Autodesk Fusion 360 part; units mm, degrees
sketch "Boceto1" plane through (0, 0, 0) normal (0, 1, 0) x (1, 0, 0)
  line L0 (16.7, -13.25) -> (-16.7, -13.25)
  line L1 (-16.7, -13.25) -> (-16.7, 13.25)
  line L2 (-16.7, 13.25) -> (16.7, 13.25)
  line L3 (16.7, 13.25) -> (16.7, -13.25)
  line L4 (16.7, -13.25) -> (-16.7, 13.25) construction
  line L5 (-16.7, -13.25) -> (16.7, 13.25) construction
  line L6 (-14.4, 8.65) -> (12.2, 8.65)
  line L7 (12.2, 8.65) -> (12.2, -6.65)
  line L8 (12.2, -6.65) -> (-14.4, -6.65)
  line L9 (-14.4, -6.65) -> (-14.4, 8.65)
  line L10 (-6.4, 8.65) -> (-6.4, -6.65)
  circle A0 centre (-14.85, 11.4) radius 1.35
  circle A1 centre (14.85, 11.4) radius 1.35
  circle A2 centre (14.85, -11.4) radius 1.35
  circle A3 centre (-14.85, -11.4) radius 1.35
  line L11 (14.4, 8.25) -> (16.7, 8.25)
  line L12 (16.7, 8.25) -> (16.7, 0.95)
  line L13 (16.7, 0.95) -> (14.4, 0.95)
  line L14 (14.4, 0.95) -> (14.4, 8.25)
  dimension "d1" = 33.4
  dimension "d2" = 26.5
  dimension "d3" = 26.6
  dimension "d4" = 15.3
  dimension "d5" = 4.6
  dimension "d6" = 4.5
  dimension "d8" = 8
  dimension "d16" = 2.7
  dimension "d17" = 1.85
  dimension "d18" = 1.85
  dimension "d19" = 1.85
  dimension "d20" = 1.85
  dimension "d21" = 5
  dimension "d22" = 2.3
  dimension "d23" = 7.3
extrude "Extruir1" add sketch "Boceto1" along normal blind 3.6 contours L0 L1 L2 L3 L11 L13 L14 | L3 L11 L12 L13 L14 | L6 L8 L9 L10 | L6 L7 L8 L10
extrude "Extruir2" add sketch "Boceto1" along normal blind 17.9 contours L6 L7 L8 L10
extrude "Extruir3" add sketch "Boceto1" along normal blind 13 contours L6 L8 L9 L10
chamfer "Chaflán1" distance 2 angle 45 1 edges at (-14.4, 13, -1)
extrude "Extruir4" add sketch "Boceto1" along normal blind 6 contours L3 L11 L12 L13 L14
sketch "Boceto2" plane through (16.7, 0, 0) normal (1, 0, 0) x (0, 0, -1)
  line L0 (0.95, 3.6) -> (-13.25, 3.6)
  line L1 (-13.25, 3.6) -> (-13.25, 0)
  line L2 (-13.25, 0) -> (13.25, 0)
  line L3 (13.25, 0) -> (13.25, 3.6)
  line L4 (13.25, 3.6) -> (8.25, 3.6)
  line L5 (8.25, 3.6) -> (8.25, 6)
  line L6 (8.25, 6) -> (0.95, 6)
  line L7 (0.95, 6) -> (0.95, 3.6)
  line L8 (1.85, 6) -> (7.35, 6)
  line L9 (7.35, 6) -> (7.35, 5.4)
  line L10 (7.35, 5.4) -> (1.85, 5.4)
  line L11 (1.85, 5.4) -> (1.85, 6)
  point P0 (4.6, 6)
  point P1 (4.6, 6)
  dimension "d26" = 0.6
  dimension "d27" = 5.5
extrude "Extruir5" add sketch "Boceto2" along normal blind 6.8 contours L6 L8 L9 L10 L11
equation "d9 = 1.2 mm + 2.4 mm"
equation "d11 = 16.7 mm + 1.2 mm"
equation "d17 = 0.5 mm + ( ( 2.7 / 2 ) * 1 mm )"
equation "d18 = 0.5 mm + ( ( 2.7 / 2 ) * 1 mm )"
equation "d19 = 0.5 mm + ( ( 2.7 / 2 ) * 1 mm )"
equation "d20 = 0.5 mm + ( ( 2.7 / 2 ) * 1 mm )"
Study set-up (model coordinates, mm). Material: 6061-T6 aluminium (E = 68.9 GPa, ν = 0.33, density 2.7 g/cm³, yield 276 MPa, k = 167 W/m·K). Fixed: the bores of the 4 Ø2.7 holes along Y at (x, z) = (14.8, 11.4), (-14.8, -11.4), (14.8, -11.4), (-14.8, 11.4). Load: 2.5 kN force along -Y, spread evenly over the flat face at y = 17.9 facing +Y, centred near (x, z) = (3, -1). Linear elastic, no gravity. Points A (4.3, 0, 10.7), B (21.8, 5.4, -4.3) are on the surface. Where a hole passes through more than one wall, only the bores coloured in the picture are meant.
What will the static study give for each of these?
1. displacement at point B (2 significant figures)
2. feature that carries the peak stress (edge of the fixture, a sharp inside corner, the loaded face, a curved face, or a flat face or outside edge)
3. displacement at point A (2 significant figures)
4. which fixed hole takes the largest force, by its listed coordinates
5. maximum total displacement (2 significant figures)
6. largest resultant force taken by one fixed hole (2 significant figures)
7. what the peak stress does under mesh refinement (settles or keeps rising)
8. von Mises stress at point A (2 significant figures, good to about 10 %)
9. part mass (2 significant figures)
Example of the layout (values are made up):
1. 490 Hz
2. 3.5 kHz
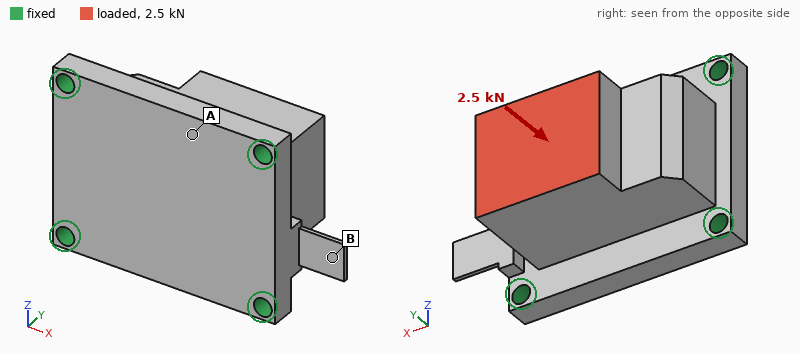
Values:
1. 6.6 µm
2. edge of the fixture
3. 14 µm
4. (14.8, -11.4)
5. 22 µm
6. 900 N
7. keeps rising
8. 31 MPa
9. 23 g
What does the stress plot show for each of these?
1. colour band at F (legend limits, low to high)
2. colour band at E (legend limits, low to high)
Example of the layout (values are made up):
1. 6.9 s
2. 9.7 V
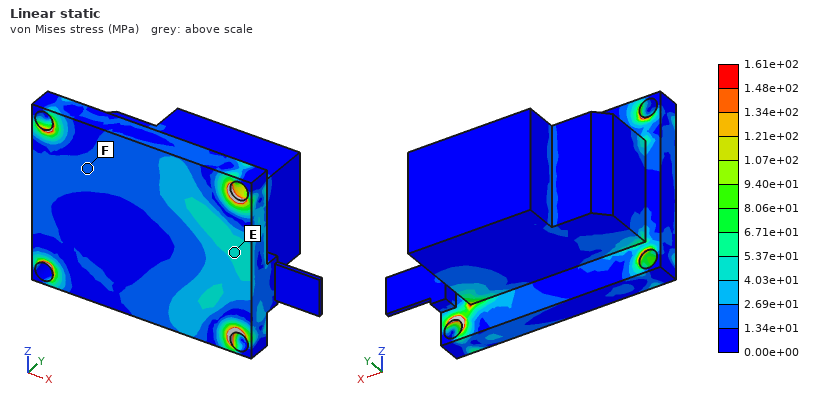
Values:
1. 1.34e+01 to 2.69e+01 MPa
2. 4.03e+01 to 5.37e+01 MPa
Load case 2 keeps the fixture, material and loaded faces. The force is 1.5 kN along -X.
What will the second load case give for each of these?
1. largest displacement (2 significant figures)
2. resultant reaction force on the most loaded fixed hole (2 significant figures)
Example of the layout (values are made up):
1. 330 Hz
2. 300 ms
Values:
1. 20 µm
2. 760 N
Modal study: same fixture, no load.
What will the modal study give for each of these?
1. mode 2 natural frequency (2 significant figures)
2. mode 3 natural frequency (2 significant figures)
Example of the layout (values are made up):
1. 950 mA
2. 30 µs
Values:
1. 14 kHz
2. 16 kHz
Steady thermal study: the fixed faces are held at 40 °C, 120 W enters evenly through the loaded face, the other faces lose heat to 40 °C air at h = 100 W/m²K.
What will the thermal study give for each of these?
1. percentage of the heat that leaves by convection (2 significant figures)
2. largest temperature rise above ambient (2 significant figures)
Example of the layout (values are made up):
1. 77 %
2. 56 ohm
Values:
1. 8.8 %
2. 71 K
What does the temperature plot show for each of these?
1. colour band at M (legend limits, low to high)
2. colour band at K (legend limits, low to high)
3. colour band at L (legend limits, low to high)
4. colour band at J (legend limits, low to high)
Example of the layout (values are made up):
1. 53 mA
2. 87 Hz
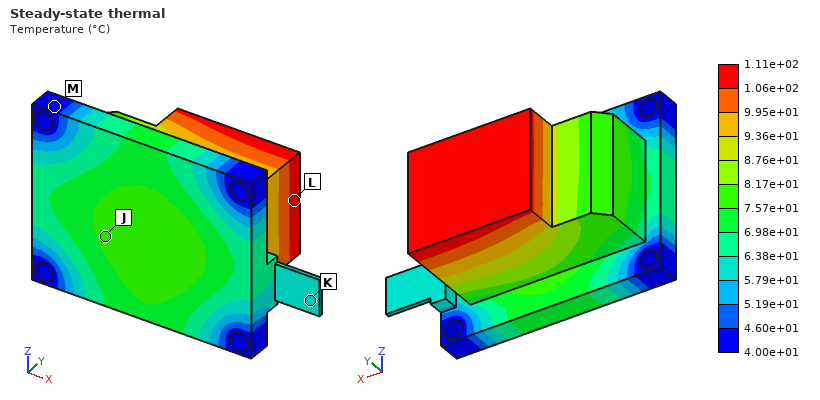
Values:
1. 4.00e+01 to 4.60e+01 °C
2. 5.79e+01 to 6.38e+01 °C
3. 1.06e+02 to 1.11e+02 °C
4. 7.57e+01 to 8.17e+01 °C
